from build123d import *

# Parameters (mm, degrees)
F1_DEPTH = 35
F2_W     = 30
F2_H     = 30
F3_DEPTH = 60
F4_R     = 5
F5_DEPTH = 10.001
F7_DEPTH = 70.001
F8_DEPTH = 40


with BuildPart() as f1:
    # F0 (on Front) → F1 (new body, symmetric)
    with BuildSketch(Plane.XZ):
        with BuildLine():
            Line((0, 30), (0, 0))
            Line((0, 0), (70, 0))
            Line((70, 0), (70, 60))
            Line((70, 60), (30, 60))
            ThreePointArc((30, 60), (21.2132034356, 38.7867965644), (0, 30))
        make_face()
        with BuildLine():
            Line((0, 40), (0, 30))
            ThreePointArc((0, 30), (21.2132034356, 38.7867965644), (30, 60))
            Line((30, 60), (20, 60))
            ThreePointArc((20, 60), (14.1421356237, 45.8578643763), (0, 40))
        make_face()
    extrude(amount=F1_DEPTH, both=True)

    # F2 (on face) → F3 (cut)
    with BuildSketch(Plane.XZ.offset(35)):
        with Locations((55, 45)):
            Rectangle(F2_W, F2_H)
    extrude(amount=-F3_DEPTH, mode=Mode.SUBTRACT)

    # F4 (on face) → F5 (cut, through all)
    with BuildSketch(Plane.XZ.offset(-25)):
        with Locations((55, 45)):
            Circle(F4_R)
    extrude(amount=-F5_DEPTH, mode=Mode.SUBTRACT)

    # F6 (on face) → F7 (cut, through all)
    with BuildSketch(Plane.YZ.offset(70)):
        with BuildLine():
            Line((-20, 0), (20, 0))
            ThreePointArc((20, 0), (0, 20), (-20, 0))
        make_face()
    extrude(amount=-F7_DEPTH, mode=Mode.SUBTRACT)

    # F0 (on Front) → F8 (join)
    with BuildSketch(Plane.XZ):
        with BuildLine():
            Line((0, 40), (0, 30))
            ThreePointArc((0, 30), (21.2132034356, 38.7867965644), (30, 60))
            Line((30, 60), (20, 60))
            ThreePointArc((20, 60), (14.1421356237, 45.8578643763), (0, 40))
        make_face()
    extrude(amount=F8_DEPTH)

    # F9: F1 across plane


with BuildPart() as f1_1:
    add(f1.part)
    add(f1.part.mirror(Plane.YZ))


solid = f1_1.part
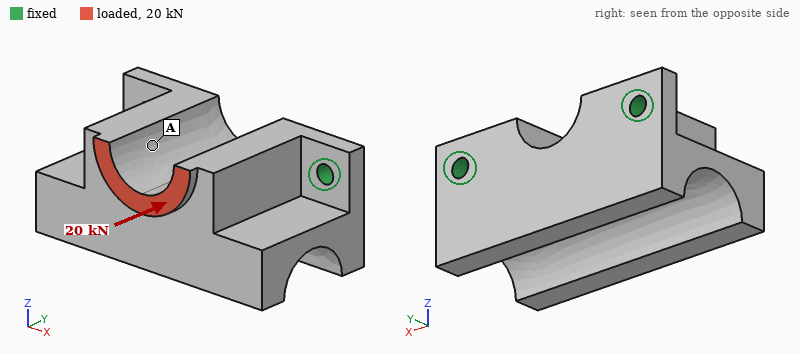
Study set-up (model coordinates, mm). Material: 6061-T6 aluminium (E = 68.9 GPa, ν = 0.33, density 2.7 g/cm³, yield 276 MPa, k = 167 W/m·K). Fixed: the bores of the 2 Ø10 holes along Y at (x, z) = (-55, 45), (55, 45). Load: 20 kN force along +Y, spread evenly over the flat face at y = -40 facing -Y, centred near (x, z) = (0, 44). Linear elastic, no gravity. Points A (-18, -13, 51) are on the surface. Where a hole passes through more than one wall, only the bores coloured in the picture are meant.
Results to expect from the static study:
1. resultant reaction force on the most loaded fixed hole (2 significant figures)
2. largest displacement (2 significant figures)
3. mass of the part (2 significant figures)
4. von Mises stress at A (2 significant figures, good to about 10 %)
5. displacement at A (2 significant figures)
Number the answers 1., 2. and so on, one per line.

1. 11 kN
2. 0.11 mm
3. 950 g
4. 20 MPa
5. 0.068 mm
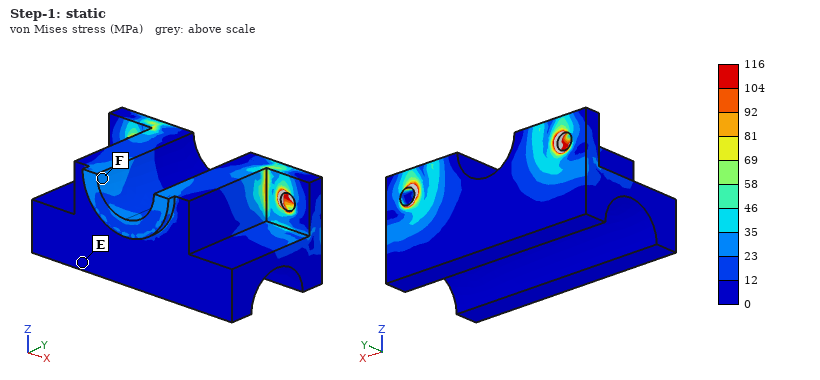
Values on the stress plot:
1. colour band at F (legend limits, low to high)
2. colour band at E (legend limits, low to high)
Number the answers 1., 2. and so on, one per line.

1. 23 to 35 MPa
2. 0 to 12 MPa
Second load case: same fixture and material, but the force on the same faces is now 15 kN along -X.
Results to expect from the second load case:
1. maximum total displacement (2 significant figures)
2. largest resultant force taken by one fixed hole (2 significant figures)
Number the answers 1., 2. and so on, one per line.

1. 0.12 mm
2. 13 kN
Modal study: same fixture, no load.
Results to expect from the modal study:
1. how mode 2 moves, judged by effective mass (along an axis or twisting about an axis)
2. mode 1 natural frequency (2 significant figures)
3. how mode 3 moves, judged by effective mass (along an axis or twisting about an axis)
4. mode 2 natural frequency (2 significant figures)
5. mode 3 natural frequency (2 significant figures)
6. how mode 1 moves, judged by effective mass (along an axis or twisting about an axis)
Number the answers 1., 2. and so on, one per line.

1. along X
2. 940 Hz
3. along X
4. 3400 Hz
5. 4000 Hz
6. along Z
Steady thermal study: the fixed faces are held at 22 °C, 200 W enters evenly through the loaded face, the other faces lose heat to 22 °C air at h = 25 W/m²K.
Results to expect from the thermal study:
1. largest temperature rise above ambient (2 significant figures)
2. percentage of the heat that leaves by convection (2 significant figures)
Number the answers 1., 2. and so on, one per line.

1. 59 K
2. 16 %
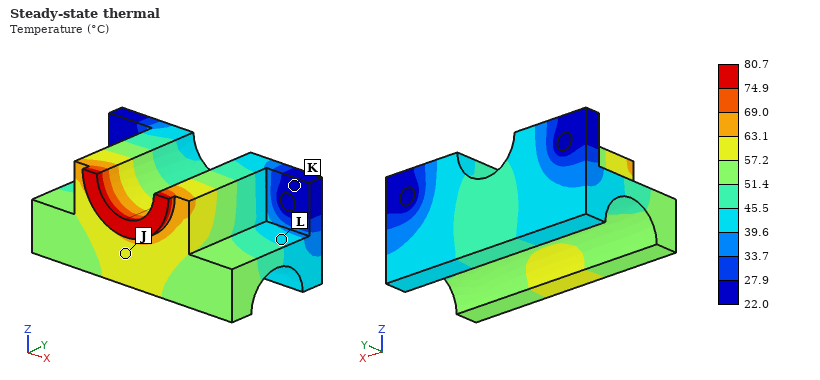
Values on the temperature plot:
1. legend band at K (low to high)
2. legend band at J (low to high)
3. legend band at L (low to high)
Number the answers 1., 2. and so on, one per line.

1. 22.0 to 27.9 °C
2. 57.2 to 63.1 °C
3. 39.6 to 45.5 °C
